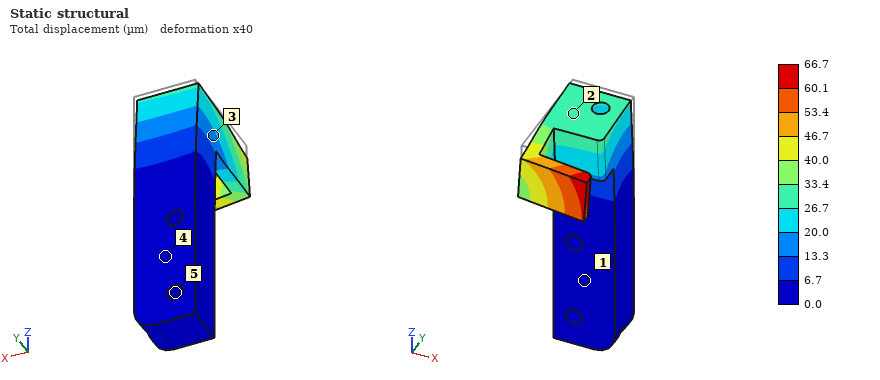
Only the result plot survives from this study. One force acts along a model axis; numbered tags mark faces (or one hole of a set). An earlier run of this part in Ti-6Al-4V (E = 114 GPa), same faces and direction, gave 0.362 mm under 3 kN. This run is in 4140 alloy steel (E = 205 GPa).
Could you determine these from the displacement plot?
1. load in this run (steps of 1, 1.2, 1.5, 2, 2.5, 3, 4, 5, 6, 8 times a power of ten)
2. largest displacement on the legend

1 kN
66.7 µm
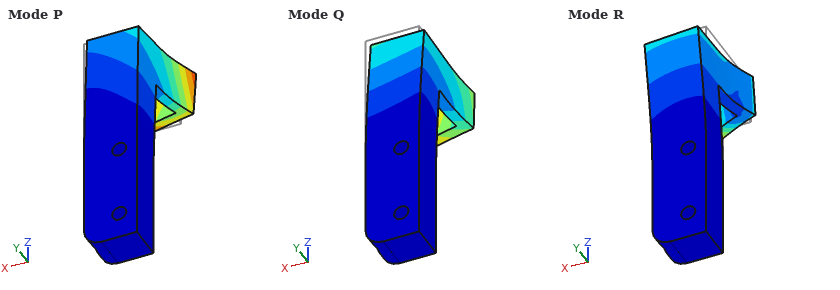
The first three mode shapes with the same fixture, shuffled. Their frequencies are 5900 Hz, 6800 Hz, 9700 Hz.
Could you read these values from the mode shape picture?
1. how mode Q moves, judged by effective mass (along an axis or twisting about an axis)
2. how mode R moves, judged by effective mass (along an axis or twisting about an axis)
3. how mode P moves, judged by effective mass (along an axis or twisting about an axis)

along Y
along X
along X
